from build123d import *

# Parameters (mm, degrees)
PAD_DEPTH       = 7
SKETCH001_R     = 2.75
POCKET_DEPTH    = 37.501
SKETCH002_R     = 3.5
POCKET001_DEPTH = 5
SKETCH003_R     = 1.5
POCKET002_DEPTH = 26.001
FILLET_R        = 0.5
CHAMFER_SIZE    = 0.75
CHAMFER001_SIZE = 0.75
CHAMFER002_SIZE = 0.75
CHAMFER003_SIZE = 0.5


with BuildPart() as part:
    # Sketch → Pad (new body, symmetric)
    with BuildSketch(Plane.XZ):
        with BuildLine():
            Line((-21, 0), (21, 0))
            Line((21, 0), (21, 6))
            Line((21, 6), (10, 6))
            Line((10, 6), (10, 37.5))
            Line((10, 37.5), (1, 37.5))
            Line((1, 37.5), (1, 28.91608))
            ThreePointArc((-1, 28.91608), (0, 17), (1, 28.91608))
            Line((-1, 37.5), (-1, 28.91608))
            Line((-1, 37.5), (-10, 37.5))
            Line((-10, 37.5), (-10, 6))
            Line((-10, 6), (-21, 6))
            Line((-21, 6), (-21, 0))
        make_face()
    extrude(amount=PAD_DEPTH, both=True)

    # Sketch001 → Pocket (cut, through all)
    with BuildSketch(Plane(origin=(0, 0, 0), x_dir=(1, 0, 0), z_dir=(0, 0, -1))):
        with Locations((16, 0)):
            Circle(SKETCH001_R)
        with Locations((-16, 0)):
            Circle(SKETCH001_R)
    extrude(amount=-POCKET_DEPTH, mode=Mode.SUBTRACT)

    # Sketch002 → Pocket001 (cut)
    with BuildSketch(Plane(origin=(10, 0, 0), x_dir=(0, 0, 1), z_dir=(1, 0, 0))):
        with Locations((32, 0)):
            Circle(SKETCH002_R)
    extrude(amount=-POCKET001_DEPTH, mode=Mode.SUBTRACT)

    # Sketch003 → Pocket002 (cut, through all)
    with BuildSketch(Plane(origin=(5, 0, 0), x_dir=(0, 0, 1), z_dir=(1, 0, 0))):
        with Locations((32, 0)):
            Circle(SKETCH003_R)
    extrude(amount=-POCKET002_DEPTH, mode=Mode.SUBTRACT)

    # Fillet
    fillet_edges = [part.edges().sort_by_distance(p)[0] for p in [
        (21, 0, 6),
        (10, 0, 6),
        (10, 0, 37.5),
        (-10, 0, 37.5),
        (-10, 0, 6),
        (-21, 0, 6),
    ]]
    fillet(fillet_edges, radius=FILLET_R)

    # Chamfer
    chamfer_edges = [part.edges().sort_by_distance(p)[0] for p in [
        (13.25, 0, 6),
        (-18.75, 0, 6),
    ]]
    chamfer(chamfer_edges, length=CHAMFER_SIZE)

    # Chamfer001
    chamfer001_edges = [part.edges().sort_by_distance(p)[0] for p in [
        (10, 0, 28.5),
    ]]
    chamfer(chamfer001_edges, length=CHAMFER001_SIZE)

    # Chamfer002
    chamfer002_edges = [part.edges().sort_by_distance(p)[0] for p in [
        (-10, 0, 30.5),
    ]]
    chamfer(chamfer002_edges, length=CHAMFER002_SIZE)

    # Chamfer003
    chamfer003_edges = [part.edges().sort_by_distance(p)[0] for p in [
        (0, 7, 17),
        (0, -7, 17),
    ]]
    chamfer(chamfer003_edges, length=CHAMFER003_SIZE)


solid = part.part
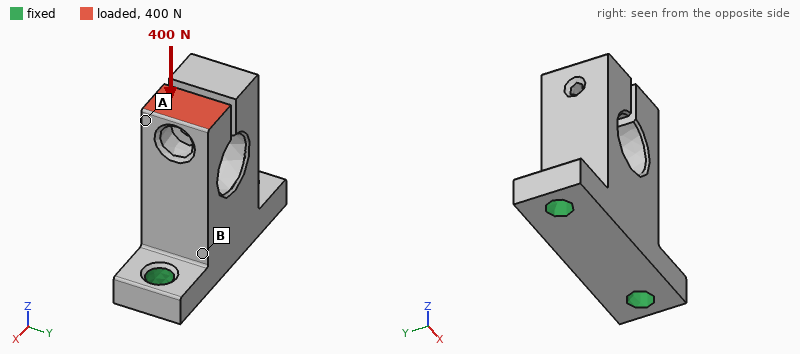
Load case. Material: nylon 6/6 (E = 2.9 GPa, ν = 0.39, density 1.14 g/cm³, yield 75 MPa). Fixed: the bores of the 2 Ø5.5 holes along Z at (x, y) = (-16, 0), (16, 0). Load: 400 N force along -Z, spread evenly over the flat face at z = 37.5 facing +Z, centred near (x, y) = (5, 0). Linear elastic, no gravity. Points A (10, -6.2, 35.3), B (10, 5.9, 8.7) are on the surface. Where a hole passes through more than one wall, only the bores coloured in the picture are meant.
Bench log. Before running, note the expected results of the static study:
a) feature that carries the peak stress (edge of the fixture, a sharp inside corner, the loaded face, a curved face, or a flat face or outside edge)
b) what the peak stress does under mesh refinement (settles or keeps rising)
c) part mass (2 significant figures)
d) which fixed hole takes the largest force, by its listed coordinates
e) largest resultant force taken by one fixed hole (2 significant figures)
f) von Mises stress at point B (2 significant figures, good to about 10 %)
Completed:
a sharp inside corner
keeps rising
11 g
(16, 0)
300 N
5.6 MPa
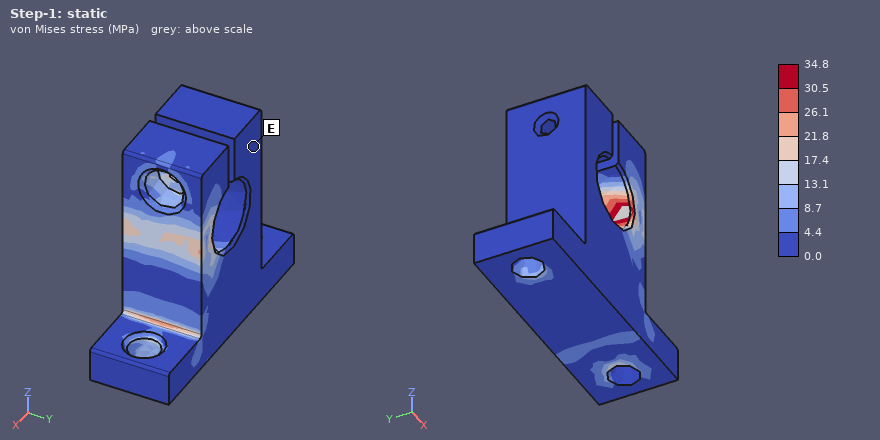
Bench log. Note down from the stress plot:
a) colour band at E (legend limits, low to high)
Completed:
0.0 to 4.4 MPa
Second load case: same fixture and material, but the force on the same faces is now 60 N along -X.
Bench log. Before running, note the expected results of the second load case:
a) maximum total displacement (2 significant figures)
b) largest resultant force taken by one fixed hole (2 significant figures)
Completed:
0.68 mm
94 N
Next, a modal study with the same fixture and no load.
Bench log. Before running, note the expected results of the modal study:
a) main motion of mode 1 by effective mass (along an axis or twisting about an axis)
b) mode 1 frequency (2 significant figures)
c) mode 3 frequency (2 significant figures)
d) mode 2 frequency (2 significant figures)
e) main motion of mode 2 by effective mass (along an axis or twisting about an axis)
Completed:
along Y
1300 Hz
1900 Hz
1800 Hz
along X
